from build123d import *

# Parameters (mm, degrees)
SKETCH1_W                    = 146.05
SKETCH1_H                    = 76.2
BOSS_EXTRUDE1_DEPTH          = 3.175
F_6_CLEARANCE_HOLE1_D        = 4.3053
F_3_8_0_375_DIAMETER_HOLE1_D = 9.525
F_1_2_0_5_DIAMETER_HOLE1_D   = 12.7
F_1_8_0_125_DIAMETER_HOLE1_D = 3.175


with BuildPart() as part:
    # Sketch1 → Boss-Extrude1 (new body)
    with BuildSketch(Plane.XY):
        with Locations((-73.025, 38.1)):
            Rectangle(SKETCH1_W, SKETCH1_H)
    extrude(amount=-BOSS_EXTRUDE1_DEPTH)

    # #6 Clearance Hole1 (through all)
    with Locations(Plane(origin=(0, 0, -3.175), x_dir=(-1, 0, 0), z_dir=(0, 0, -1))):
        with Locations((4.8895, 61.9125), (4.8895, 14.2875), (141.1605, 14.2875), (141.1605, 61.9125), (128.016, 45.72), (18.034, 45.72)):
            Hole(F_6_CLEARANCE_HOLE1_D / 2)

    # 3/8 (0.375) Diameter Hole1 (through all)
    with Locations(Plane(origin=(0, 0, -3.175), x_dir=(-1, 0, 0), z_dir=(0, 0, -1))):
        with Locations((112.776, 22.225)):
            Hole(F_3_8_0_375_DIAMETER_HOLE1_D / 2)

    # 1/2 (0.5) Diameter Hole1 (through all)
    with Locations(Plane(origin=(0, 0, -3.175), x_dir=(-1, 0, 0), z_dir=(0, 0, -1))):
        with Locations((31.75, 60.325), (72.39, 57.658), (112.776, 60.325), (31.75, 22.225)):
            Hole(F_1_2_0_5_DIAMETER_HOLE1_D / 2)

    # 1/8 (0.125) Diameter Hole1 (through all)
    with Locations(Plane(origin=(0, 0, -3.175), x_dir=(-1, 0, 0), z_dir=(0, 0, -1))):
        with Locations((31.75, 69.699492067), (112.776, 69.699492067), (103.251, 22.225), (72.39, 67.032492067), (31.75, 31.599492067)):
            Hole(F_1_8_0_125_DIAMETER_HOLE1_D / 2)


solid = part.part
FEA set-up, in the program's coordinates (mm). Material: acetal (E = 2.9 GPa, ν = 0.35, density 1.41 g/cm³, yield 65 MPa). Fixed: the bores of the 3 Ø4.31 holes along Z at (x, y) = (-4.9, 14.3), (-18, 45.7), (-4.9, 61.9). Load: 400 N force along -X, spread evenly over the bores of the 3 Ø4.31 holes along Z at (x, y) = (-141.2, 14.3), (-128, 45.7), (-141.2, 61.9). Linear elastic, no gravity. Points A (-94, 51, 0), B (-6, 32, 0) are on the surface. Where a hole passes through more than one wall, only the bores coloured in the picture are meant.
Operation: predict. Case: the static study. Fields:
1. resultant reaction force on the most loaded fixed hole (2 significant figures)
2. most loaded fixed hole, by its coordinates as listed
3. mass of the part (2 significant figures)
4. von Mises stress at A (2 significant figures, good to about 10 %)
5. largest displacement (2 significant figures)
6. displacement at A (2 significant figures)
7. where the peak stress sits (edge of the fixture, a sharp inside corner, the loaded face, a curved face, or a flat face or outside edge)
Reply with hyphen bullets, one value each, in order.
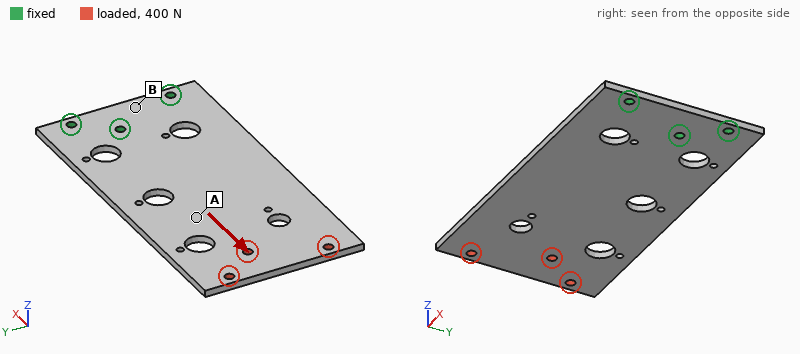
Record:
- 180 N
- (-18, 45.7)
- 47 g
- 1.8 MPa
- 0.13 mm
- 0.074 mm
- a curved face
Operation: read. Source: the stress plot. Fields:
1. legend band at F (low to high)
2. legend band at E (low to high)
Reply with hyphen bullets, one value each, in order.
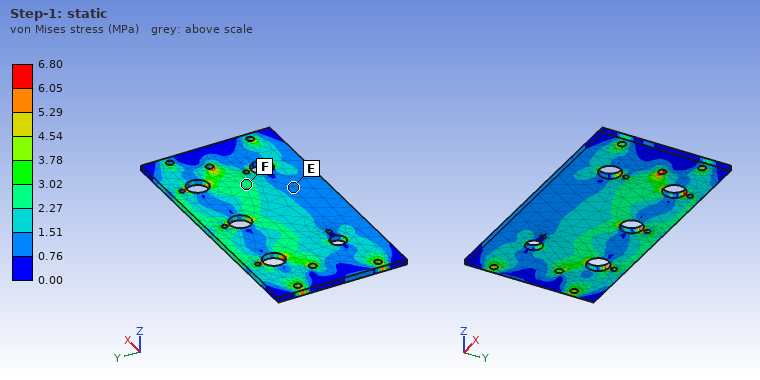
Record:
- 2.27 to 3.02 MPa
- 0.76 to 1.51 MPa
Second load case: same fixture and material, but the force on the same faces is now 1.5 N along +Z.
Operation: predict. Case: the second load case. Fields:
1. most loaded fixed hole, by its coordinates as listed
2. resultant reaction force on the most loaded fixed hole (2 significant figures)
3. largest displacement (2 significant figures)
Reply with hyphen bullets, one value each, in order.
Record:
- (-18, 45.7)
- 5.8 N
- 2.0 mm
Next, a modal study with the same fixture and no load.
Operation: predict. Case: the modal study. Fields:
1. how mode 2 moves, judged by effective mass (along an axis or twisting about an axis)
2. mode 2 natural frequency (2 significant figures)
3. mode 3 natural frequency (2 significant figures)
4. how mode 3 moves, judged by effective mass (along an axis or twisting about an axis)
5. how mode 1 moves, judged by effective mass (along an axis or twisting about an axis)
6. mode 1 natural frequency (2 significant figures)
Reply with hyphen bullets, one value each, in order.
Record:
- twisting about X
- 150 Hz
- 250 Hz
- along Z
- along Z
- 41 Hz
